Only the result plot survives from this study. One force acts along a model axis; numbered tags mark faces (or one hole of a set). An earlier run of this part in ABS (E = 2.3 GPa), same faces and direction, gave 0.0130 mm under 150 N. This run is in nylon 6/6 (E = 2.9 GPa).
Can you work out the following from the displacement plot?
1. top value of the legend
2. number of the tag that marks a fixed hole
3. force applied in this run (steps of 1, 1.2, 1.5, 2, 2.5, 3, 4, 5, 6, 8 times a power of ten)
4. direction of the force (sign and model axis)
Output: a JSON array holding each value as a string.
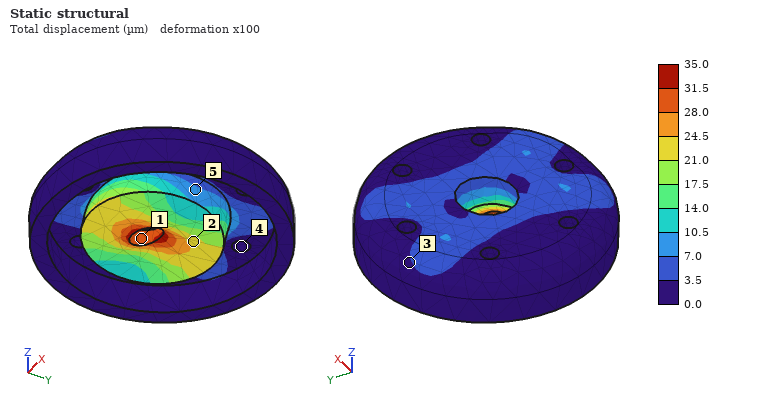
["35.0 µm", "4", "500 N", "-Y"]
